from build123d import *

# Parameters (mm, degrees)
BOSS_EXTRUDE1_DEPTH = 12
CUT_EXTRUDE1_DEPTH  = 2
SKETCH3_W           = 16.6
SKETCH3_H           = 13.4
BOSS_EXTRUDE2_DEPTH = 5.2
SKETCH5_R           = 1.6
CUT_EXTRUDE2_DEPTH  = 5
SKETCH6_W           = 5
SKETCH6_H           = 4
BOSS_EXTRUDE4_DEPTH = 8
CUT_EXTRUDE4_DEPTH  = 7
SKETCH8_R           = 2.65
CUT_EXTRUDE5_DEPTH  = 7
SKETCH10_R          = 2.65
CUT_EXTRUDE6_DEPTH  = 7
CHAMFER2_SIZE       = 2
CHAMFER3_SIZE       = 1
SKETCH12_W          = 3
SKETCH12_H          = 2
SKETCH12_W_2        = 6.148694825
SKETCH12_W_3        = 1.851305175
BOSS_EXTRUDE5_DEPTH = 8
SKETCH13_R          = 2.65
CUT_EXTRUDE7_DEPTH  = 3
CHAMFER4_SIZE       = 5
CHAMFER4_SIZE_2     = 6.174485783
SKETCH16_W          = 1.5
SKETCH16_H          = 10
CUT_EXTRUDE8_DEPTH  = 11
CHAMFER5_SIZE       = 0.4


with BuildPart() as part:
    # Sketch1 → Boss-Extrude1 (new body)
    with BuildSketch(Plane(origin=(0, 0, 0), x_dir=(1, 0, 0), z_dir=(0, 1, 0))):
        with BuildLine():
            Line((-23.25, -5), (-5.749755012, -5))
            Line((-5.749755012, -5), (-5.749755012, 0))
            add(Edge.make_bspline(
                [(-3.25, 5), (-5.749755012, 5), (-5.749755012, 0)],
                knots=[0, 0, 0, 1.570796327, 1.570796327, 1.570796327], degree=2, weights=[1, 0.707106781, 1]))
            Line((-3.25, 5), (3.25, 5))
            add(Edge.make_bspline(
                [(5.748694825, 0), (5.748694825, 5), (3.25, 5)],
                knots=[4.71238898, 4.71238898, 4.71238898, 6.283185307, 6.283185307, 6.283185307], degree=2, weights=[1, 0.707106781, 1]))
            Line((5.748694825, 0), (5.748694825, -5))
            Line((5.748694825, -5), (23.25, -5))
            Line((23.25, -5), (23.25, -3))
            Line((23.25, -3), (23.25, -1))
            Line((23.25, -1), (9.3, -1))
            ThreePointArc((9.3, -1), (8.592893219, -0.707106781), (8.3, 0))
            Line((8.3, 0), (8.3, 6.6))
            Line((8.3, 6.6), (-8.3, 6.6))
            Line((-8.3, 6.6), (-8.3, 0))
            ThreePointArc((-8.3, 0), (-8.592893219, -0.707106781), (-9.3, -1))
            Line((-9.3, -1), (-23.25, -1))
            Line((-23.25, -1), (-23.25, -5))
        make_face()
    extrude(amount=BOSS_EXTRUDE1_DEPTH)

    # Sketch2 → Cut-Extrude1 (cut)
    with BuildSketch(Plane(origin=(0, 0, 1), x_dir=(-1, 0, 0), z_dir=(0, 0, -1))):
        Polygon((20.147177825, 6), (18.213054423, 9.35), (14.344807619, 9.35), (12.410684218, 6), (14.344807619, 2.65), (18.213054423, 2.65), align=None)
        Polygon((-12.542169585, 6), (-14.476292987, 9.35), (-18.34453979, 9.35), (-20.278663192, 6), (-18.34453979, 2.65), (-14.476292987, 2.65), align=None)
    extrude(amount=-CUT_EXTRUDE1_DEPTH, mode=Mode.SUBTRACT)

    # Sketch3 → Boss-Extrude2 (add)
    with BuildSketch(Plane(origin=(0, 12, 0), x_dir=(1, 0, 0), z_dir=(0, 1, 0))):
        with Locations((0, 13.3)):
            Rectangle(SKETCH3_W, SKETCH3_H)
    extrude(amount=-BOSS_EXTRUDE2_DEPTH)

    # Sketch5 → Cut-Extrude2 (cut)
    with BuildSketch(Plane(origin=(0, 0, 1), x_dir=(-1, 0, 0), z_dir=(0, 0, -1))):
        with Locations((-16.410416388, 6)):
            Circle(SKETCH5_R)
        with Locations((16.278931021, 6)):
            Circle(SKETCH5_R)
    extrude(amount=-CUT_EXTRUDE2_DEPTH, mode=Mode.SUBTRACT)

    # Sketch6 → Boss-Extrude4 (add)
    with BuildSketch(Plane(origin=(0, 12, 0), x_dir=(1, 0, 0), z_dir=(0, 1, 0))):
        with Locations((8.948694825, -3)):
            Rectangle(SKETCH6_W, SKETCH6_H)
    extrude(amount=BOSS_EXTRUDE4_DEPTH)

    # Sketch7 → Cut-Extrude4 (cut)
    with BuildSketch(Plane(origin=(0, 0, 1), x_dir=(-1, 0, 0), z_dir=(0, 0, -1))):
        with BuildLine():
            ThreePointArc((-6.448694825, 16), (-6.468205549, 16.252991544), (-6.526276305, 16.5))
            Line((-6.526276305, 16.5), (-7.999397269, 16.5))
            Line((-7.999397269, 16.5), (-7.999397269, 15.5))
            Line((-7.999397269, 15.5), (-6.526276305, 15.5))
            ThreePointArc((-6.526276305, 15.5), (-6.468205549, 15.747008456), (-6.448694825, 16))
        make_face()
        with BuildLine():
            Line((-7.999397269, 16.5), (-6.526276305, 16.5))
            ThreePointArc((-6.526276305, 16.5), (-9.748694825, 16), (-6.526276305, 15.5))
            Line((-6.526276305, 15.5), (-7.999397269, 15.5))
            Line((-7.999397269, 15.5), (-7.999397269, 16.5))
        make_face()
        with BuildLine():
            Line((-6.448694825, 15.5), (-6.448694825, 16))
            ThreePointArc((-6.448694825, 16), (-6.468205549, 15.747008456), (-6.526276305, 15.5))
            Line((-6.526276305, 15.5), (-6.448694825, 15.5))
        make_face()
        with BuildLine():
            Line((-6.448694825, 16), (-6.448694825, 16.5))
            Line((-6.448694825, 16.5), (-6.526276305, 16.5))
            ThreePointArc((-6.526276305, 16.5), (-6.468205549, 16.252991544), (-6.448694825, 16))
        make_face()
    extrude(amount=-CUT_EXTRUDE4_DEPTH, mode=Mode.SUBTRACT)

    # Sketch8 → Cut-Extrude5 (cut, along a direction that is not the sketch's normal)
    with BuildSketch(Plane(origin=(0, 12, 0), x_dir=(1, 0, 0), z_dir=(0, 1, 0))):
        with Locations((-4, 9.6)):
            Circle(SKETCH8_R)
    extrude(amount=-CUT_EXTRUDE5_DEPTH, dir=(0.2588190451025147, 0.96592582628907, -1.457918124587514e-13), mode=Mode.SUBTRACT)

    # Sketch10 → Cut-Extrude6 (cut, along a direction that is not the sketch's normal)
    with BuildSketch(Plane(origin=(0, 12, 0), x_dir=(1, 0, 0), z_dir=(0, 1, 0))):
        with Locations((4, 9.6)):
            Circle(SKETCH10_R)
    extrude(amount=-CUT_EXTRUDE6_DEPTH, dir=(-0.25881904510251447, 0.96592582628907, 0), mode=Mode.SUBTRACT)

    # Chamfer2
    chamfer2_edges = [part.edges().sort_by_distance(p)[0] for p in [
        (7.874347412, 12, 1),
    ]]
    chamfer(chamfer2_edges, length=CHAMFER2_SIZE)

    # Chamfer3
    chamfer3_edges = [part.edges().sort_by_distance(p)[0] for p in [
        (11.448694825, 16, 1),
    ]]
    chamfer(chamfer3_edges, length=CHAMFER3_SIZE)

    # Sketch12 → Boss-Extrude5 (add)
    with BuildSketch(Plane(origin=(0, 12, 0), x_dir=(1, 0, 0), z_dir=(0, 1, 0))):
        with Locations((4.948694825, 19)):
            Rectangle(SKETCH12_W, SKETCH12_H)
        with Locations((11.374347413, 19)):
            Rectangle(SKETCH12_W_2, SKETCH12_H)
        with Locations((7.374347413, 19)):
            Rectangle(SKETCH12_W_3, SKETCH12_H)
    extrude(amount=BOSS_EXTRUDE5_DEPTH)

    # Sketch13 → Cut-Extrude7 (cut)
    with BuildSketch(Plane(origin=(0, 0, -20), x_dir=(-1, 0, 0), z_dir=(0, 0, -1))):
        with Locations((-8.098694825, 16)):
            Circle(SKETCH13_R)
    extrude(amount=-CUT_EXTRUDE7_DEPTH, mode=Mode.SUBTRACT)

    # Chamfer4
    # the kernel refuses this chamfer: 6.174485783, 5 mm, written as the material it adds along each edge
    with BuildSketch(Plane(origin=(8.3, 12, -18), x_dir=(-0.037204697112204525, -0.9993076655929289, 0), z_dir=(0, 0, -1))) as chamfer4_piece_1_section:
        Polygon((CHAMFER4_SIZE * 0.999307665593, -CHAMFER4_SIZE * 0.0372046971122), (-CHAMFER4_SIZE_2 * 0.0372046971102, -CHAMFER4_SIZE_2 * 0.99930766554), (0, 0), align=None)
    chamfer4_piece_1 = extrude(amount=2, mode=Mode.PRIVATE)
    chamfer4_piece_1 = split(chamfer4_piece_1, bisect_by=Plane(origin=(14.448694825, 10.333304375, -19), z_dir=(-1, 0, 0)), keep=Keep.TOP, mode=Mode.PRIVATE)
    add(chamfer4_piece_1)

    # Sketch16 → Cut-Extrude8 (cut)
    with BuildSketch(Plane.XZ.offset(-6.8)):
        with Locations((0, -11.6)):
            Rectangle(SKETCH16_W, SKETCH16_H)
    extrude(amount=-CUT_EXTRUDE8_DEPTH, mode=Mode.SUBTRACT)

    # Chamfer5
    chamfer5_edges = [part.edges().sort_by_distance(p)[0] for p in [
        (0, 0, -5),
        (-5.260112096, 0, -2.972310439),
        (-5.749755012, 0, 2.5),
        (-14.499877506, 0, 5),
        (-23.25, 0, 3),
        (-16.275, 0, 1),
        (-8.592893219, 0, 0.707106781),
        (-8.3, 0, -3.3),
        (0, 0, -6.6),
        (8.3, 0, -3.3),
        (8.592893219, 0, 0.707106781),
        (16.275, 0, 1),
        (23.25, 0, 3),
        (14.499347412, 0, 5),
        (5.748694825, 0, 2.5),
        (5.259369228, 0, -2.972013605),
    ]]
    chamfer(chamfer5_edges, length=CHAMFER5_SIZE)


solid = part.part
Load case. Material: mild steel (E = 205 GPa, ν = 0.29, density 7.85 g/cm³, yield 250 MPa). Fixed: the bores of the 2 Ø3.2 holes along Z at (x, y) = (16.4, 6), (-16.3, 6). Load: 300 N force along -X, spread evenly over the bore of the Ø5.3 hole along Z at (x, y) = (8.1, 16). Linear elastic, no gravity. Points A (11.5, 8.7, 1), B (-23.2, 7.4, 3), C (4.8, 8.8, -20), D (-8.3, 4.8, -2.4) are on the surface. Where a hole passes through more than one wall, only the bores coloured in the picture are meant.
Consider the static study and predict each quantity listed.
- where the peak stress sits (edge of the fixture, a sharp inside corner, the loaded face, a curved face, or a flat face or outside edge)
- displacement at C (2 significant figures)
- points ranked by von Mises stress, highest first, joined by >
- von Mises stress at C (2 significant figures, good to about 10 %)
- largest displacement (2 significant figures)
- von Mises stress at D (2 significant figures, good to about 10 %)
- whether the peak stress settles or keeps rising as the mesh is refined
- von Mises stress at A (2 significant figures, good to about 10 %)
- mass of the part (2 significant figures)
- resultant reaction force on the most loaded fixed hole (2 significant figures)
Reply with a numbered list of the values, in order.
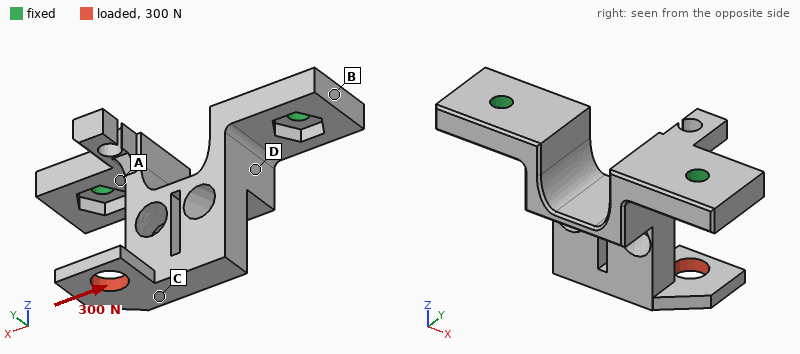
1. edge of the fixture
2. 20 µm
3. D > C > A > B
4. 38 MPa
5. 61 µm
6. 55 MPa
7. keeps rising
8. 22 MPa
9. 26 g
10. 330 N
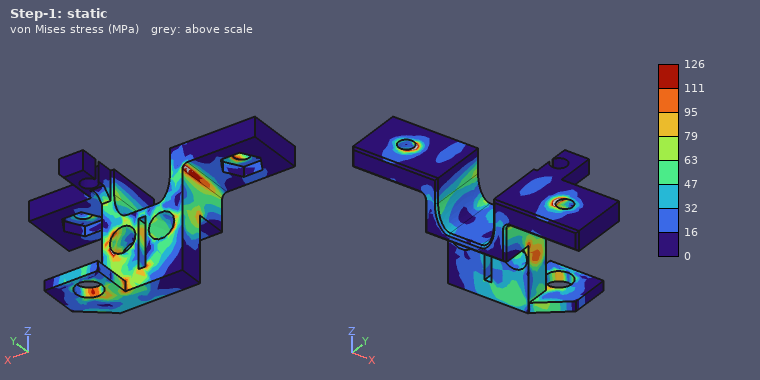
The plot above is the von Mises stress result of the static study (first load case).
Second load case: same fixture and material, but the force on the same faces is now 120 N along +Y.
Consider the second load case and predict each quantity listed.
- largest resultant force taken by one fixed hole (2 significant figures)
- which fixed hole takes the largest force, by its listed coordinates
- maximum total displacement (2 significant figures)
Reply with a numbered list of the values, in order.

1. 84 N
2. (16.4, 6)
3. 65 µm
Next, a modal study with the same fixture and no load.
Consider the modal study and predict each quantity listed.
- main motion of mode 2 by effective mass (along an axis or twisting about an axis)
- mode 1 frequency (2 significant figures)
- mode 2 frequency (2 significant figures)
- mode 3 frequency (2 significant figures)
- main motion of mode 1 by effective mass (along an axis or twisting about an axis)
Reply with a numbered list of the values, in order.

1. along X
2. 3400 Hz
3. 7500 Hz
4. 9200 Hz
5. along Y
